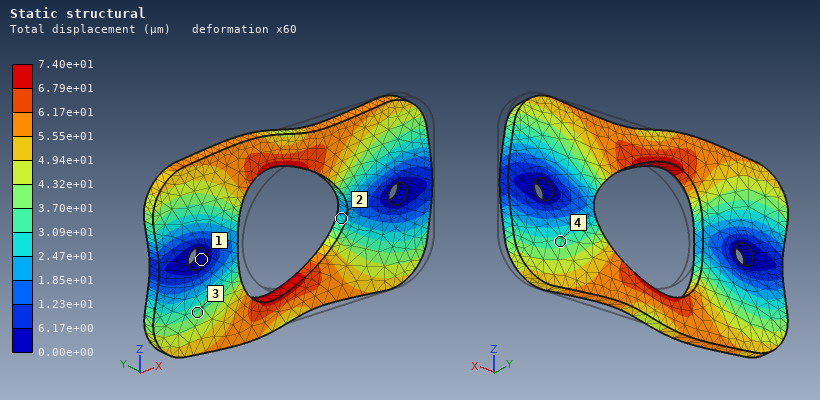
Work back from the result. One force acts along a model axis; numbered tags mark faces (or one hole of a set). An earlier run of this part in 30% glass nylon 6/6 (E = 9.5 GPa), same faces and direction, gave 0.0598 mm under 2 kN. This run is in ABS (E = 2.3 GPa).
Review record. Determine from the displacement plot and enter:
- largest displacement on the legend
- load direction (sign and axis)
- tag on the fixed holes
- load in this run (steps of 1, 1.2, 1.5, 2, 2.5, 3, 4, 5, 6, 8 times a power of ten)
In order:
7.40e+01 µm
-X
1
600 N
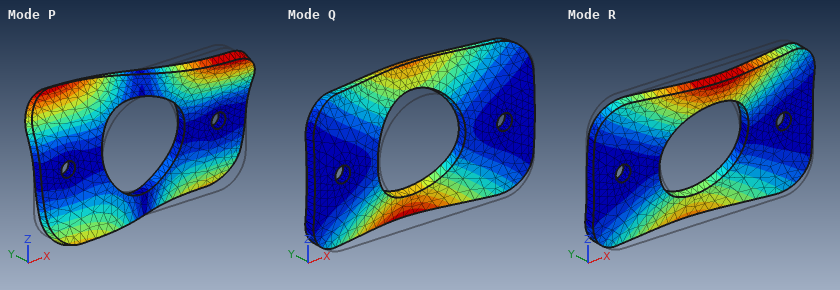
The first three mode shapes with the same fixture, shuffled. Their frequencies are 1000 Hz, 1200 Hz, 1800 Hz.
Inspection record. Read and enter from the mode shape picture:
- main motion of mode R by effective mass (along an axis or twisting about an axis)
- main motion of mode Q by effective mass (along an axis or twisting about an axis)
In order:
twisting about X
along Y
